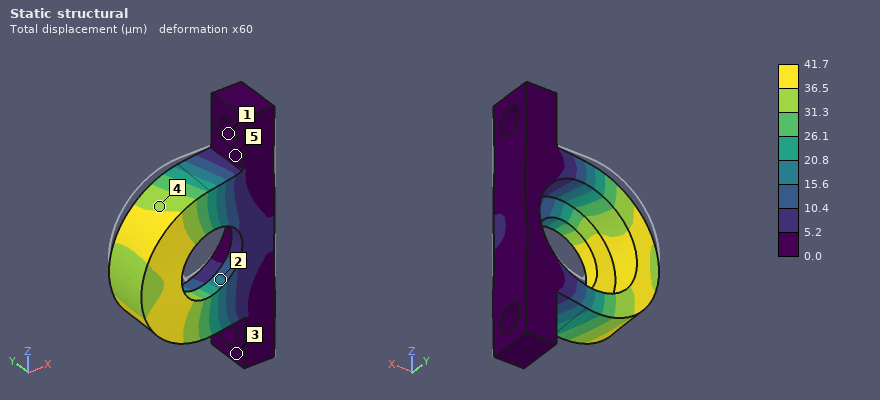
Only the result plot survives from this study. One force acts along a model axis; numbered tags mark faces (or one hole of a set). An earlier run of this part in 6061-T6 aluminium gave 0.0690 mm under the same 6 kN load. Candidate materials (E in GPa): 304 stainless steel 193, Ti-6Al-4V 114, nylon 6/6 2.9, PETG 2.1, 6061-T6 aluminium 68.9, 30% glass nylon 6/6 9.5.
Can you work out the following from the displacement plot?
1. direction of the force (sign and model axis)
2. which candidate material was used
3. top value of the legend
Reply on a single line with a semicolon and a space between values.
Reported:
-Z; Ti-6Al-4V; 41.7 µm
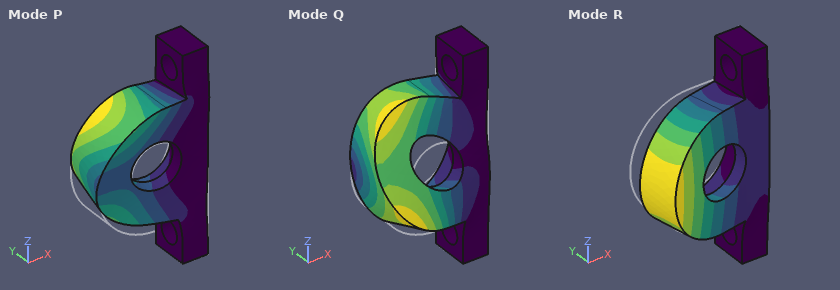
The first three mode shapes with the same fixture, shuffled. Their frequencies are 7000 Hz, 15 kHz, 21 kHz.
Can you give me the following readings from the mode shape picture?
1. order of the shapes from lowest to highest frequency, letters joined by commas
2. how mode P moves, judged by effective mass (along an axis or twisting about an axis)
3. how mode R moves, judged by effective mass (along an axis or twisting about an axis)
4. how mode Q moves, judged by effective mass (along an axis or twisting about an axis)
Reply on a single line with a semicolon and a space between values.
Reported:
R, P, Q; along Z; along Y; along Z
